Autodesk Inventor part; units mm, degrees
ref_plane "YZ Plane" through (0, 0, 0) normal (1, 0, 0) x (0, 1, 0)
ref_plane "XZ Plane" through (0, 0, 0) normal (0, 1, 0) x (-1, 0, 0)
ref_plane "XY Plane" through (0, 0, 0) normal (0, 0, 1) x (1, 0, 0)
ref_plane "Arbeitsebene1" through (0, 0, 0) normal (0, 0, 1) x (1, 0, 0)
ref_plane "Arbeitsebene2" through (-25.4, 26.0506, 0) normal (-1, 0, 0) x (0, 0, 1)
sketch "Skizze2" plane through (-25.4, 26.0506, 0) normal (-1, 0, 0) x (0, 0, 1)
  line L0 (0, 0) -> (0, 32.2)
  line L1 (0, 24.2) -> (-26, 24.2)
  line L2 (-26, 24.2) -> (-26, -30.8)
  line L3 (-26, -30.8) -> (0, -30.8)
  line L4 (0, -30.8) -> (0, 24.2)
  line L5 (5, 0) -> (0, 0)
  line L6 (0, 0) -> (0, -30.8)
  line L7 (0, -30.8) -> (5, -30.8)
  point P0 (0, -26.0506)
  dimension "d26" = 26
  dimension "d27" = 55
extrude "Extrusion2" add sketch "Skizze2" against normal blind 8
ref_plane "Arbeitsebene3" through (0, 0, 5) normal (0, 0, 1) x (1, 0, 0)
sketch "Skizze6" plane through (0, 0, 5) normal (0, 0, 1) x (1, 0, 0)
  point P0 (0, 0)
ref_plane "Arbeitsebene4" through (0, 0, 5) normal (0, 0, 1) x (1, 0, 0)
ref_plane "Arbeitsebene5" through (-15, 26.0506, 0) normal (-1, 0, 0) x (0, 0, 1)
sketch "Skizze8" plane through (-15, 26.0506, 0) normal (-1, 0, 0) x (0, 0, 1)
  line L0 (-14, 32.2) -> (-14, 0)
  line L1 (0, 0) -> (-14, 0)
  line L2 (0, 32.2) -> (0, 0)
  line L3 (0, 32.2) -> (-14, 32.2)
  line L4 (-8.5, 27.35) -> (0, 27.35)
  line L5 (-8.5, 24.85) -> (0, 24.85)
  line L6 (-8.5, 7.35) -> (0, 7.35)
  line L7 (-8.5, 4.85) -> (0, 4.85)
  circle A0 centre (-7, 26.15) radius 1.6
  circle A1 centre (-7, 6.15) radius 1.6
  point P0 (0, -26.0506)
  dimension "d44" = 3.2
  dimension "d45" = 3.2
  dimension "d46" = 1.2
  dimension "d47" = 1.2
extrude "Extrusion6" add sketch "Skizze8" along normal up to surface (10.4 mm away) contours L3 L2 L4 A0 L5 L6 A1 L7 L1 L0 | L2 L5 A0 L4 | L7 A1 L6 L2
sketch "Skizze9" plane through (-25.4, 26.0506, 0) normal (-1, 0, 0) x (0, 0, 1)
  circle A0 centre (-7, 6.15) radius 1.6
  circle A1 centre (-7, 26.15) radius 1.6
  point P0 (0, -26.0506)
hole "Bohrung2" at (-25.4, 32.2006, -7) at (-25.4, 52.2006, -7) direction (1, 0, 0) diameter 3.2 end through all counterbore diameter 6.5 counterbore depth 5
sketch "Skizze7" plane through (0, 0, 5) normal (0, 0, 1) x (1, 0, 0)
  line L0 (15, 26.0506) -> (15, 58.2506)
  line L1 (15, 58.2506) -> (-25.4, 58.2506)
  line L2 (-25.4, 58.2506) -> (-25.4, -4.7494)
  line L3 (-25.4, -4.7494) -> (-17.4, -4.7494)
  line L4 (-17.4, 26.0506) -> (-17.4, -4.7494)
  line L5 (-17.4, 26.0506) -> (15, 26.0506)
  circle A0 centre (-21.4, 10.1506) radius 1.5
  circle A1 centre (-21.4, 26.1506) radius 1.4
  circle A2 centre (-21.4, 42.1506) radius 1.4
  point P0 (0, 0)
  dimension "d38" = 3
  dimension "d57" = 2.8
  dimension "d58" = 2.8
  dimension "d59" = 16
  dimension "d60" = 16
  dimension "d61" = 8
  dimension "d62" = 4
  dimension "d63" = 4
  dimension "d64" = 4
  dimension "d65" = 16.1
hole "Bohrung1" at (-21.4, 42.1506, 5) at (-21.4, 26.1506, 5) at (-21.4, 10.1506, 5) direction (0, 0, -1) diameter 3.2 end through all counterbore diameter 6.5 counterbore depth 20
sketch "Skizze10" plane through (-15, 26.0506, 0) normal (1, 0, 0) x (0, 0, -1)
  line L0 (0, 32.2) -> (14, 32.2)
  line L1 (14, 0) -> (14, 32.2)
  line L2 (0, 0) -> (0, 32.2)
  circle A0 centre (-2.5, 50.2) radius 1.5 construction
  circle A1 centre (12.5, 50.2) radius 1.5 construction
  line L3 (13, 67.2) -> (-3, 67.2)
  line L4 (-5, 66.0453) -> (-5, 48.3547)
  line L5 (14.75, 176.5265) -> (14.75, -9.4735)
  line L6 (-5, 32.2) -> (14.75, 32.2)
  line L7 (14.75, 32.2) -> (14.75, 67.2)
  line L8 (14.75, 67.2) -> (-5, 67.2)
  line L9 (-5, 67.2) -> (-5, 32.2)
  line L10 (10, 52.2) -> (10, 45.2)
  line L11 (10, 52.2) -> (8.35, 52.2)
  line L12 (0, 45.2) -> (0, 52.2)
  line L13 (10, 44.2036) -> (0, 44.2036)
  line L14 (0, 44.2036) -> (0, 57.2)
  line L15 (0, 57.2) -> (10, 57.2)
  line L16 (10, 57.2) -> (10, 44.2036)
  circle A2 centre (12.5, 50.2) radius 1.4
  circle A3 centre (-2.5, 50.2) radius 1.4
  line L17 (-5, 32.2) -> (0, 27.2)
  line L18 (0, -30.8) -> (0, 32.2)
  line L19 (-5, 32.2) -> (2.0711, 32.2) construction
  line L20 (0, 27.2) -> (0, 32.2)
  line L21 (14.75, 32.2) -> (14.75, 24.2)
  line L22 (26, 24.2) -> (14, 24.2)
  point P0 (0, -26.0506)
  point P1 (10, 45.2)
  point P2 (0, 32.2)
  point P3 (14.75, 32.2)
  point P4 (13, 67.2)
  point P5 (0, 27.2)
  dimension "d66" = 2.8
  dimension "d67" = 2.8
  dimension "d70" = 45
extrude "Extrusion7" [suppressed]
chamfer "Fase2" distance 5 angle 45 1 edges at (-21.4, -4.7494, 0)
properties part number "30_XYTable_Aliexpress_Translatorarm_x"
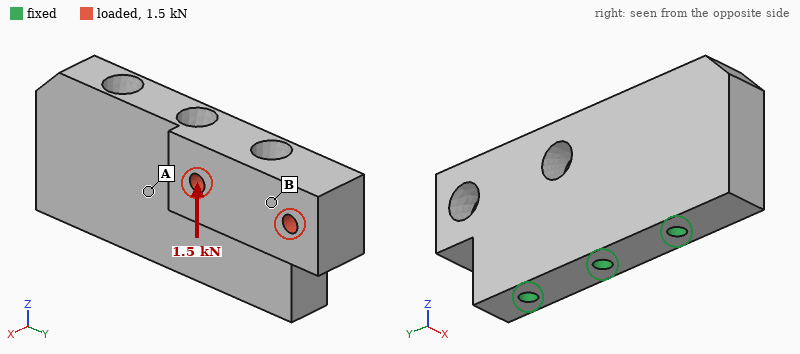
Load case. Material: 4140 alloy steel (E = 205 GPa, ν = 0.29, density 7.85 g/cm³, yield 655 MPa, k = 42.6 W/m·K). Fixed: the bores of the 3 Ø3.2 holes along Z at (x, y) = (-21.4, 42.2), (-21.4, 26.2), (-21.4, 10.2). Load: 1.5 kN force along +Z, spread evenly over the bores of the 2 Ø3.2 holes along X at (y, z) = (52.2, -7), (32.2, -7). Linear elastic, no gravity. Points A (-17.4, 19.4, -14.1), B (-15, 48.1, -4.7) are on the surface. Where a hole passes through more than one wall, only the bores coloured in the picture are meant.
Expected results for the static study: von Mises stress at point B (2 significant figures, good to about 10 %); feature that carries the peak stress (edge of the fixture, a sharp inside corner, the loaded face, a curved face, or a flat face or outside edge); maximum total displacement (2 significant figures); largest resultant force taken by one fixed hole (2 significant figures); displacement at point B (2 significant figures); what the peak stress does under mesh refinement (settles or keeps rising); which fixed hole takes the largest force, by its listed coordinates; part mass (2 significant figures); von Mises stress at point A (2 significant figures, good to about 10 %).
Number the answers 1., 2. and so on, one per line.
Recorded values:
1. 15 MPa
2. edge of the fixture
3. 7.1 µm
4. 1.2 kN
5. 4.4 µm
6. keeps rising
7. (-21.4, 42.2)
8. 87 g
9. 5.3 MPa
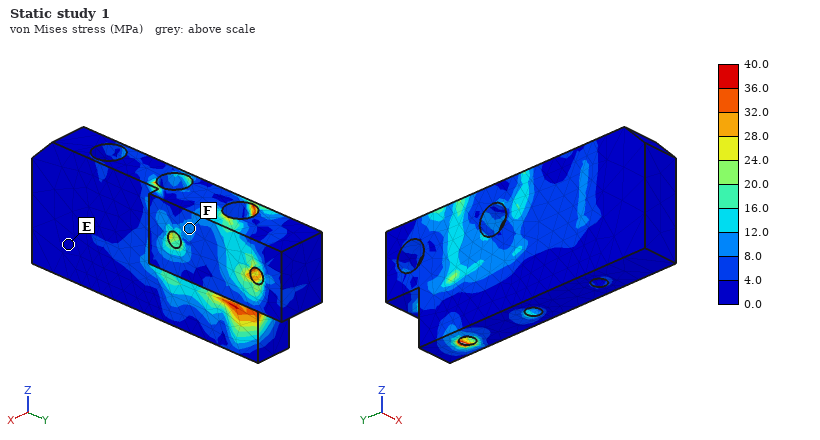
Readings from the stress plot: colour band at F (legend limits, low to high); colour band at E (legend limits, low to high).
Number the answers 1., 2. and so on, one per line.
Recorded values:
1. 8.0 to 12.0 MPa
2. 0.0 to 4.0 MPa
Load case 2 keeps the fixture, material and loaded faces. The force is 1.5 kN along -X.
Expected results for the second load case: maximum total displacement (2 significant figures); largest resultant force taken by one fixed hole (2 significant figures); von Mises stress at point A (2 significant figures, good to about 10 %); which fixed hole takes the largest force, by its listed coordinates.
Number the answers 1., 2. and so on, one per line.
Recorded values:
1. 19 µm
2. 1.3 kN
3. 15 MPa
4. (-21.4, 42.2)
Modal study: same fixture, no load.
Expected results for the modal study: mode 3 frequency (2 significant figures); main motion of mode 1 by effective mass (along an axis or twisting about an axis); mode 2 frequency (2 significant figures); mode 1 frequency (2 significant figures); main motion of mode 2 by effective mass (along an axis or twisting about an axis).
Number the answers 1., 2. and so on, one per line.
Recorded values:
1. 17 kHz
2. along X
3. 13 kHz
4. 11 kHz
5. along X
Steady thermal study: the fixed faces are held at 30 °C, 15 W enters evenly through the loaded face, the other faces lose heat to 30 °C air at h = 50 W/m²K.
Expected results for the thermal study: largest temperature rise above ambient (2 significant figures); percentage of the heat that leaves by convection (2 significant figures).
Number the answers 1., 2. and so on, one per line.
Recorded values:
1. 32 K
2. 16 %
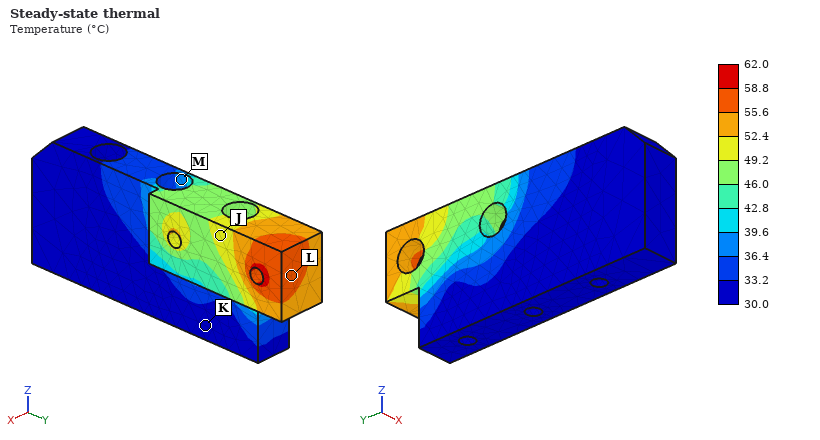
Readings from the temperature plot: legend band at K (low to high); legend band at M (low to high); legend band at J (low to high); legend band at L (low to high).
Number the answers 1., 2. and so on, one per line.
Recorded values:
1. 30.0 to 33.2 °C
2. 36.4 to 39.6 °C
3. 49.2 to 52.4 °C
4. 55.6 to 58.8 °C
